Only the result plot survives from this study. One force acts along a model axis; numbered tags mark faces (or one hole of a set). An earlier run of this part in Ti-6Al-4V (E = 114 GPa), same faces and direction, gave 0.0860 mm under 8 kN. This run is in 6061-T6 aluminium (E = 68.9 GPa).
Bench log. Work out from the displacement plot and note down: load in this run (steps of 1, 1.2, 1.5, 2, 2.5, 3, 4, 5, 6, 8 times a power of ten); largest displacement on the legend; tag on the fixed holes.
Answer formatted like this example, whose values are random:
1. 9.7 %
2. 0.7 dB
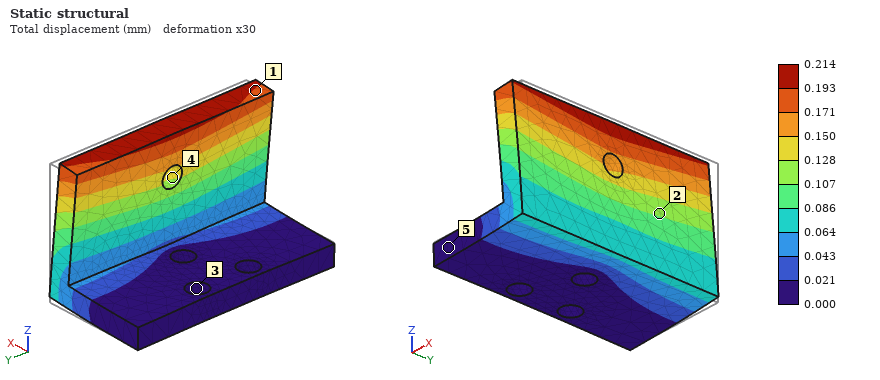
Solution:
1. 12 kN
2. 0.214 mm
3. 3
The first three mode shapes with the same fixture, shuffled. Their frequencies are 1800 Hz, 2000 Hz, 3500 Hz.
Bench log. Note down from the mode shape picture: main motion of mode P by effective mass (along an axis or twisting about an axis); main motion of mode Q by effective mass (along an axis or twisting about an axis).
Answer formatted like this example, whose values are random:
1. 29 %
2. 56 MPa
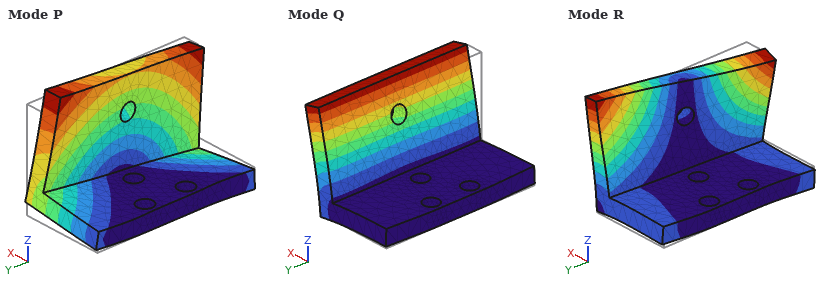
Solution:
1. along Y
2. along X
